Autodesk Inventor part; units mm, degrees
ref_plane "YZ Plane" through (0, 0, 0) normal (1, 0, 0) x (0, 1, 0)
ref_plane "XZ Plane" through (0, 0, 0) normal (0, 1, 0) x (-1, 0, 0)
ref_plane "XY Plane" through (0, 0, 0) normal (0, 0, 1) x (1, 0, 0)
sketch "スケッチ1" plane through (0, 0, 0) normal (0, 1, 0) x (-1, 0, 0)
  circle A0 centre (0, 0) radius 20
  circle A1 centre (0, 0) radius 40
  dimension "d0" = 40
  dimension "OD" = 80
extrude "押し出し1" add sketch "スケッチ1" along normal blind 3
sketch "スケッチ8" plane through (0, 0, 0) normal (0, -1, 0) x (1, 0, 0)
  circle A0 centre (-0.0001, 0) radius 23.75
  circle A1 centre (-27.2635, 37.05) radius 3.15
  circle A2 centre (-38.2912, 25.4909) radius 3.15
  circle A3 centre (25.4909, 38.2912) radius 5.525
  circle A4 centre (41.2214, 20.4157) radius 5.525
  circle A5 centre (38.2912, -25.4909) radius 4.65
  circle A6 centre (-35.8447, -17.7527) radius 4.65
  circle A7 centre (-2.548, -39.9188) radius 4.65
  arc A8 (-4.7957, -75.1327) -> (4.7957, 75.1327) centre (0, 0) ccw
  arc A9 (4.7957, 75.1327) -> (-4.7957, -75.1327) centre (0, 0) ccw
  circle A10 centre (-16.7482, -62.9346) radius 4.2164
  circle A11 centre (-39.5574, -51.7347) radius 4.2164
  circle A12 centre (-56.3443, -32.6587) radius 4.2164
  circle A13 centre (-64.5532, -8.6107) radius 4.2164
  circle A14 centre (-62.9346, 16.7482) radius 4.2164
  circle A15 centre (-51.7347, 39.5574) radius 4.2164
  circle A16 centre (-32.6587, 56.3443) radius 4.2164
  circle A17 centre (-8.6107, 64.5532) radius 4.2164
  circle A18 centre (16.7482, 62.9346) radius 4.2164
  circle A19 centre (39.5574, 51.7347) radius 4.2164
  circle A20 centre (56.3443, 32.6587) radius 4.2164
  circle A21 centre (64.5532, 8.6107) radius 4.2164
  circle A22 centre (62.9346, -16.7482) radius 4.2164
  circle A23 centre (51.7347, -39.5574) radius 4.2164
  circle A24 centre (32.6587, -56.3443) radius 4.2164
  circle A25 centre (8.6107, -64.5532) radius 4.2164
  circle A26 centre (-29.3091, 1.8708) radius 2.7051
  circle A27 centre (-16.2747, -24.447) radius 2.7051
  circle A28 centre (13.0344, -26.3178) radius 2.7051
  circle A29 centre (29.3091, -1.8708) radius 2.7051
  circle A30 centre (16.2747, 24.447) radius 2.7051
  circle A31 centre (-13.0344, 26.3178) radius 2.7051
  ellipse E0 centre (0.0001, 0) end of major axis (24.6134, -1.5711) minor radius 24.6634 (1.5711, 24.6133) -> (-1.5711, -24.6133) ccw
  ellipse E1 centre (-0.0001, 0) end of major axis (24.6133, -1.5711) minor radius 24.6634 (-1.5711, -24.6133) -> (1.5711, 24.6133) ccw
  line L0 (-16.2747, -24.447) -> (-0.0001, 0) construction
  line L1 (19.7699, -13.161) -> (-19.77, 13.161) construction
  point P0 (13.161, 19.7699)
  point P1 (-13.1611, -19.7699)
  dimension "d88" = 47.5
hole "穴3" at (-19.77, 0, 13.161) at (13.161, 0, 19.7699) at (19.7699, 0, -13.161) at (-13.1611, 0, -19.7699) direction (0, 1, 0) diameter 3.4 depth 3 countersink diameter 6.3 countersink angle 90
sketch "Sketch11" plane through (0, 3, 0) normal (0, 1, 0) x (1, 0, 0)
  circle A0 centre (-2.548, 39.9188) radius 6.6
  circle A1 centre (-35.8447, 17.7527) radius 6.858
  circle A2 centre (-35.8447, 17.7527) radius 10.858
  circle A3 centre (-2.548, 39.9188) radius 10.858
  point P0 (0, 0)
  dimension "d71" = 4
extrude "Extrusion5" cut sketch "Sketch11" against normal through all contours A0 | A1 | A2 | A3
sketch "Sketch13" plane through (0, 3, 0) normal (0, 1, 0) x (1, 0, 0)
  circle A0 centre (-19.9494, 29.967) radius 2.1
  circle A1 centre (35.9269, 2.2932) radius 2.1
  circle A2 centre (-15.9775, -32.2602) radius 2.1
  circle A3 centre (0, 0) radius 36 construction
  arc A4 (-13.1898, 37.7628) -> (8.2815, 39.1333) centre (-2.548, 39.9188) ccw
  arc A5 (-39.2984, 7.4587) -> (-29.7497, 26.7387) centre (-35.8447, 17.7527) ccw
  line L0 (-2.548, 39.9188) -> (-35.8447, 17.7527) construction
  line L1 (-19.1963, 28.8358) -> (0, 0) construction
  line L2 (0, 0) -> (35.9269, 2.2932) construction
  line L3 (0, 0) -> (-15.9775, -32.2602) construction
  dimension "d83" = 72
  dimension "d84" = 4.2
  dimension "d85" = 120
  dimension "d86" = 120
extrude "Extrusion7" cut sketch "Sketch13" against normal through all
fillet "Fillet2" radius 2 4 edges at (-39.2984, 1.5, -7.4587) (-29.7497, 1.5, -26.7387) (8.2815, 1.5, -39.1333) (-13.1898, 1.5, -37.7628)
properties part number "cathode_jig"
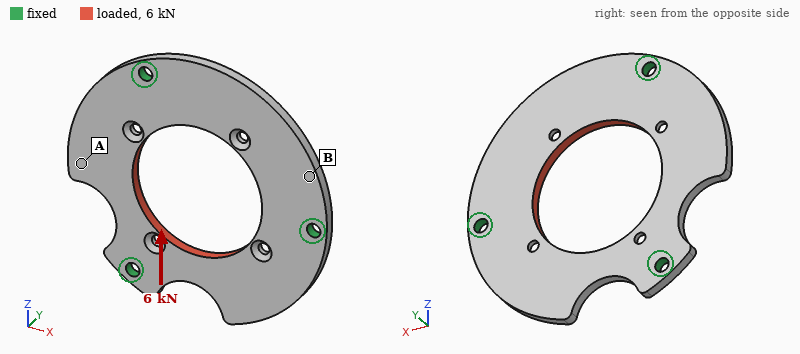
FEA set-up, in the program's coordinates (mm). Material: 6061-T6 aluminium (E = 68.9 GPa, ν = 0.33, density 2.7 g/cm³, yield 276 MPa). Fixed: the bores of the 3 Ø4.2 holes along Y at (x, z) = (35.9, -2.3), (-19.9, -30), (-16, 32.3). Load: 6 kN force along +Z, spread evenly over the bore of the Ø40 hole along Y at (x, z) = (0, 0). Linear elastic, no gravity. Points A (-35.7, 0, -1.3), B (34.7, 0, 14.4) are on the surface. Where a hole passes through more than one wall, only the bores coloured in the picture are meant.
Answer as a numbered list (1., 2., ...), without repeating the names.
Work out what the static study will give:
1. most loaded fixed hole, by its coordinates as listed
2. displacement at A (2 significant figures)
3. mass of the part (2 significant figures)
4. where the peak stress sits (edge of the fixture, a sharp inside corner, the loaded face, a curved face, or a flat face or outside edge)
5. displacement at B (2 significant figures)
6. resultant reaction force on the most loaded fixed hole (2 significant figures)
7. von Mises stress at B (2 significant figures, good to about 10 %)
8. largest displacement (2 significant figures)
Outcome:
1. (35.9, -2.3)
2. 22 µm
3. 27 g
4. edge of the fixture
5. 14 µm
6. 2.4 kN
7. 34 MPa
8. 52 µm
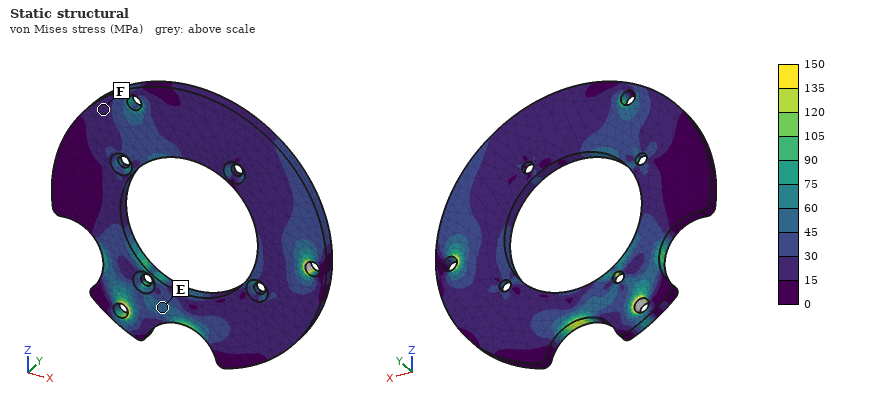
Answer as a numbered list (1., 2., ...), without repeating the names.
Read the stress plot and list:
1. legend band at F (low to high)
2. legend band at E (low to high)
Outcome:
1. 15 to 30 MPa
2. 45 to 60 MPa
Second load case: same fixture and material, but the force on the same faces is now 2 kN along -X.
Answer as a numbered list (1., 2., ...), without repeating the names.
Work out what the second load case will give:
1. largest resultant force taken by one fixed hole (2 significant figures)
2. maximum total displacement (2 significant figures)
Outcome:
1. 760 N
2. 22 µm
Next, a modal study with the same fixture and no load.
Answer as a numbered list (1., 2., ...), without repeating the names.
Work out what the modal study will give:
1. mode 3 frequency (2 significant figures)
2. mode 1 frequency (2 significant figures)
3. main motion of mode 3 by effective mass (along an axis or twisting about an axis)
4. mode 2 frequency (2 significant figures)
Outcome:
1. 3100 Hz
2. 2700 Hz
3. along Y
4. 2700 Hz
